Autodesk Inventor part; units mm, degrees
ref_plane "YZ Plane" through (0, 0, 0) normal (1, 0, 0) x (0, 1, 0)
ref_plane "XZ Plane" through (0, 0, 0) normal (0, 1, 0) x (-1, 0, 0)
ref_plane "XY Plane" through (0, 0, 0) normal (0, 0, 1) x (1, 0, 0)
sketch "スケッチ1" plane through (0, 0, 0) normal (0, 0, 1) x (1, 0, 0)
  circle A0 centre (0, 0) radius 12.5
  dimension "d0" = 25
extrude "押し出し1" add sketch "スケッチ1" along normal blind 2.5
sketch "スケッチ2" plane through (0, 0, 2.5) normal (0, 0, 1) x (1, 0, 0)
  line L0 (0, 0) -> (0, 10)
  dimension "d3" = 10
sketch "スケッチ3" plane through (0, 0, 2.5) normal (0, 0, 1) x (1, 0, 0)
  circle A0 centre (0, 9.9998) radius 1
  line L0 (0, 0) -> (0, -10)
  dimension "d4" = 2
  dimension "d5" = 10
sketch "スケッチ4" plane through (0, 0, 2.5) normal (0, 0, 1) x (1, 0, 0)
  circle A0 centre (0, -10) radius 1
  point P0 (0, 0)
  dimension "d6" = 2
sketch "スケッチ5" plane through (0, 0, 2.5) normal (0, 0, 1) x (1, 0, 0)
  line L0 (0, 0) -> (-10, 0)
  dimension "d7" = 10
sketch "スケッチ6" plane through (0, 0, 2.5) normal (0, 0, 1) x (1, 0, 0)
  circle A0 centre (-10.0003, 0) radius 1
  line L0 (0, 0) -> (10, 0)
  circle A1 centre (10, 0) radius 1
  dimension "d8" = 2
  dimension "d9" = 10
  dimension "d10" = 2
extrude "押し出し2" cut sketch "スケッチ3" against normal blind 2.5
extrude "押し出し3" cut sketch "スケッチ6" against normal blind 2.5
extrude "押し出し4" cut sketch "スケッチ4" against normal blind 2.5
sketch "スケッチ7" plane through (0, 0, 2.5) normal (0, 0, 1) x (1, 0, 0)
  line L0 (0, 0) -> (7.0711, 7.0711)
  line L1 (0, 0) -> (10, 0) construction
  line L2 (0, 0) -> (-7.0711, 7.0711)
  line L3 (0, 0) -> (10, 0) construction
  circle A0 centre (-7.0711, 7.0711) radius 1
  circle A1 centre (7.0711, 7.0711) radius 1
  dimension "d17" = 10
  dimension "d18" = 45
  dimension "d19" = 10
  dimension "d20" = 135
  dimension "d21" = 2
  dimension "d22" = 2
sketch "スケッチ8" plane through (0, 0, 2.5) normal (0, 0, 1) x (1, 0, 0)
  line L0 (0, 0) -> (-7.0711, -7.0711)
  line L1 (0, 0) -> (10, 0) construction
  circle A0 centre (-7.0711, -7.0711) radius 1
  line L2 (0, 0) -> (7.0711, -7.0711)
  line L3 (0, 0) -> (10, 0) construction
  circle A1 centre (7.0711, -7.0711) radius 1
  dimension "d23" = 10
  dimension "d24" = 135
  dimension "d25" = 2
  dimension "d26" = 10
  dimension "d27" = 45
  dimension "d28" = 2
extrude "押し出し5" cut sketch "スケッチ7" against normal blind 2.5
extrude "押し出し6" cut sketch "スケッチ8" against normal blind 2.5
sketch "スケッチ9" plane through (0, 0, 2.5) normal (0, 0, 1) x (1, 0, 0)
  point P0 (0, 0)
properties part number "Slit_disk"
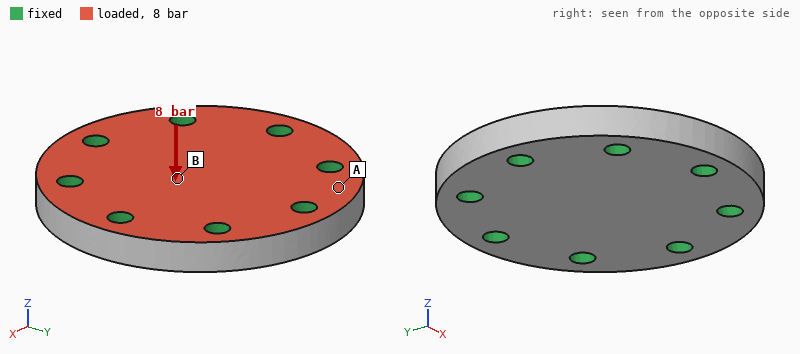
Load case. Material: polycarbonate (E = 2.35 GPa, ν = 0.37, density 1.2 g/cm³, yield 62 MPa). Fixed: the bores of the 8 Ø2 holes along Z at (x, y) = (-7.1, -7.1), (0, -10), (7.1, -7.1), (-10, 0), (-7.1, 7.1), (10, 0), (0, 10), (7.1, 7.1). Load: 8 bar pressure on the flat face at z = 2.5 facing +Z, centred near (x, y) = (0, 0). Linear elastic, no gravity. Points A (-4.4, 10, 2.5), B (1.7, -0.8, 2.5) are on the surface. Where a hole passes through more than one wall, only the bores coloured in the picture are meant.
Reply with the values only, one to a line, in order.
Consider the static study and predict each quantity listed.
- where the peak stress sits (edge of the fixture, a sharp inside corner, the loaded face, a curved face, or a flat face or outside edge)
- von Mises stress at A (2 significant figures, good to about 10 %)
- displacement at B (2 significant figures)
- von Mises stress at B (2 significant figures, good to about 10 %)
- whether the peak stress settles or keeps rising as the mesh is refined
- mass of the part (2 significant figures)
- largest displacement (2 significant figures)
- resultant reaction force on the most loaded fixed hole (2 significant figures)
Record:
edge of the fixture
2.2 MPa
41 µm
5.4 MPa
keeps rising
1.4 g
43 µm
47 N
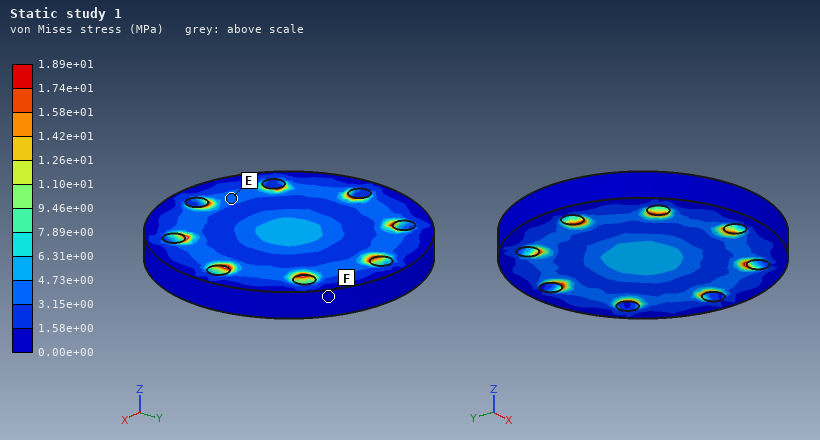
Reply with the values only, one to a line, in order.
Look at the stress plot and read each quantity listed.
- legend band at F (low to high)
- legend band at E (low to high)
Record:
0.00e+00 to 1.58e+00 MPa
3.15e+00 to 4.73e+00 MPa
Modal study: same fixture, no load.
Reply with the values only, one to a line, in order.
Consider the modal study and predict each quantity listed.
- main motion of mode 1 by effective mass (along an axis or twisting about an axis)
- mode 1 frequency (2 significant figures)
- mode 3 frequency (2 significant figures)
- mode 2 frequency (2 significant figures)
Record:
along Z
15 kHz
28 kHz
28 kHz
